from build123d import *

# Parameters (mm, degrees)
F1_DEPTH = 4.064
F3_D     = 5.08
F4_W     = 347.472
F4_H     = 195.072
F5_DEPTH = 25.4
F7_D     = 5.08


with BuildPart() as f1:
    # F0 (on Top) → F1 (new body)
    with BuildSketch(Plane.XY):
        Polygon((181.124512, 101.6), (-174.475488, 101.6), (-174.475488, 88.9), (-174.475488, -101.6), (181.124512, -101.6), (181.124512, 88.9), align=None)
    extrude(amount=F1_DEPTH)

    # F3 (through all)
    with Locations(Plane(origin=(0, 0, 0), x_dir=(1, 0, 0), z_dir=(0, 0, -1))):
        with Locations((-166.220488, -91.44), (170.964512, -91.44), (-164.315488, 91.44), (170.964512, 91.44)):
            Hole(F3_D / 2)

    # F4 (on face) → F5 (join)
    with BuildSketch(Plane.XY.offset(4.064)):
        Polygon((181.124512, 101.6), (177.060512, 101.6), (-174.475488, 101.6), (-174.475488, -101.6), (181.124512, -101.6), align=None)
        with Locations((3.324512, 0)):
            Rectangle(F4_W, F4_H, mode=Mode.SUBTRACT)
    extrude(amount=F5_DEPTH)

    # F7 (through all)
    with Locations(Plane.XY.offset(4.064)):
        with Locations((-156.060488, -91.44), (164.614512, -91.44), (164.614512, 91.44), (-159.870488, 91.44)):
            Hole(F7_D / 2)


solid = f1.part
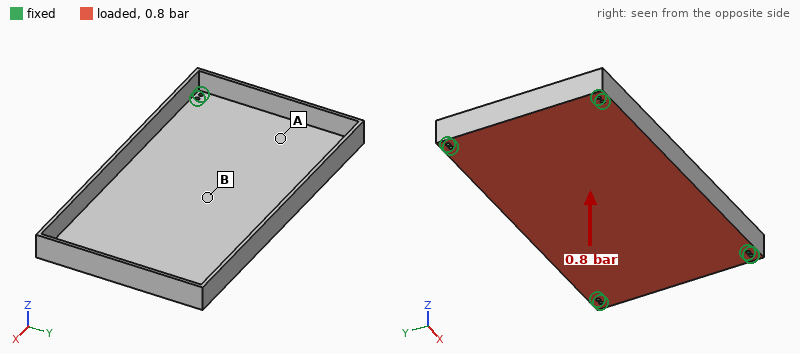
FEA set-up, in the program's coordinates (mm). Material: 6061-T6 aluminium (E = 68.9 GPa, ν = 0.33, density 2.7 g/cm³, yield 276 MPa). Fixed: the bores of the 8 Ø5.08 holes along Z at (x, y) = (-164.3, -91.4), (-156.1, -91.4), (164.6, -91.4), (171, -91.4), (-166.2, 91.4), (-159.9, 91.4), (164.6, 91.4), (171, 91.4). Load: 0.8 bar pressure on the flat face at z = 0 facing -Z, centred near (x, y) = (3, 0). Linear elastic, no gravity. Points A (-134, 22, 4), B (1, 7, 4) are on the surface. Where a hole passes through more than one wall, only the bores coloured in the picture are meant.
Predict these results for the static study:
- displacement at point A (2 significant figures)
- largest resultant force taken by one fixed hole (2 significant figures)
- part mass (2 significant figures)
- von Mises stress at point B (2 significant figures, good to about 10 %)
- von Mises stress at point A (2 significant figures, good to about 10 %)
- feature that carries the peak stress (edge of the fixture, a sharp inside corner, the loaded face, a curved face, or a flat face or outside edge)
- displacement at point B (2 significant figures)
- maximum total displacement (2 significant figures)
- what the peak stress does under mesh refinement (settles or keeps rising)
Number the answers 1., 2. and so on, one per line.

1. 0.75 mm
2. 3.1 kN
3. 1.1 kg
4. 74 MPa
5. 33 MPa
6. edge of the fixture
7. 2.4 mm
8. 2.4 mm
9. keeps rising
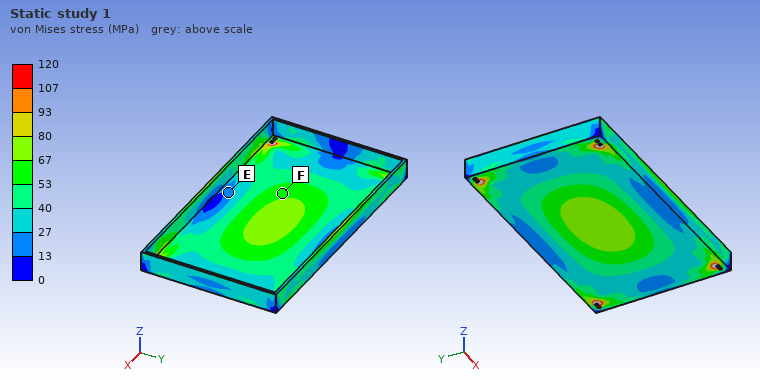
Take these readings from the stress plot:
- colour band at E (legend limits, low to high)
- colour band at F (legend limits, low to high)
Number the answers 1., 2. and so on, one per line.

1. 13 to 27 MPa
2. 53 to 67 MPa
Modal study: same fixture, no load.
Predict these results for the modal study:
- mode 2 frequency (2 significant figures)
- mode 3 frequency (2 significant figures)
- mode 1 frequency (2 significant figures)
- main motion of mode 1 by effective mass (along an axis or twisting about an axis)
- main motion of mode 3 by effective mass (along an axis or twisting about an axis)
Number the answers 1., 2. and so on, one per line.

1. 640 Hz
2. 760 Hz
3. 340 Hz
4. along Z
5. twisting about X
